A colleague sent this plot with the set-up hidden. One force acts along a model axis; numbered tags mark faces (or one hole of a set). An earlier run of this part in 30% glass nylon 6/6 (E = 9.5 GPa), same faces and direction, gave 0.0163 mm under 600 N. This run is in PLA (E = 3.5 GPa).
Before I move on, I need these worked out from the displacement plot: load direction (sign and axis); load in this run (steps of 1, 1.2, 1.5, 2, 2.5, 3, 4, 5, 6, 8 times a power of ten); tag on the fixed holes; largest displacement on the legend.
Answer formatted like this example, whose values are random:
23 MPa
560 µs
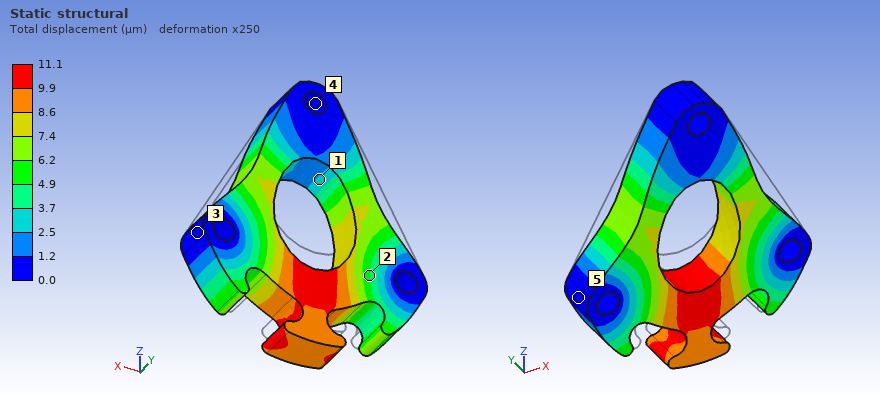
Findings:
-Z
150 N
4
11.1 µm
